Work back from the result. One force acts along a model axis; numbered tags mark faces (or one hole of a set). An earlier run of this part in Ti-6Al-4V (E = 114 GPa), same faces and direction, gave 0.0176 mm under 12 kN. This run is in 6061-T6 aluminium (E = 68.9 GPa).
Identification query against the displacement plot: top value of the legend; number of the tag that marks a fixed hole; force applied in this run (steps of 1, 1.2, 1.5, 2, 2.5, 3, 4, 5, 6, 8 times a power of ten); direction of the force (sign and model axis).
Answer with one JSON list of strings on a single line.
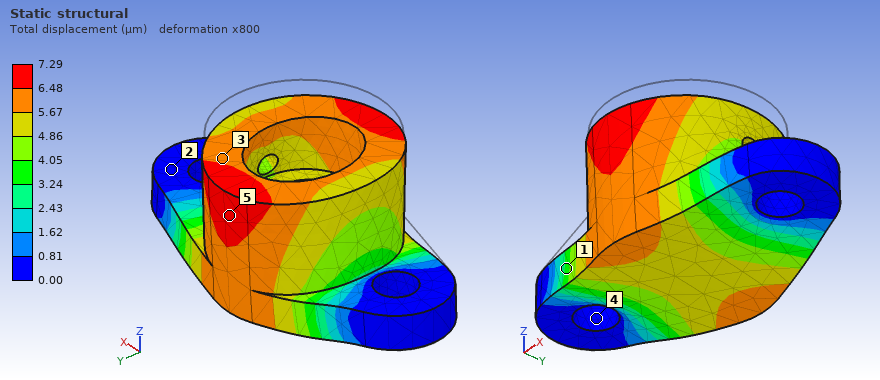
["7.29 µm", "4", "3 kN", "-Z"]
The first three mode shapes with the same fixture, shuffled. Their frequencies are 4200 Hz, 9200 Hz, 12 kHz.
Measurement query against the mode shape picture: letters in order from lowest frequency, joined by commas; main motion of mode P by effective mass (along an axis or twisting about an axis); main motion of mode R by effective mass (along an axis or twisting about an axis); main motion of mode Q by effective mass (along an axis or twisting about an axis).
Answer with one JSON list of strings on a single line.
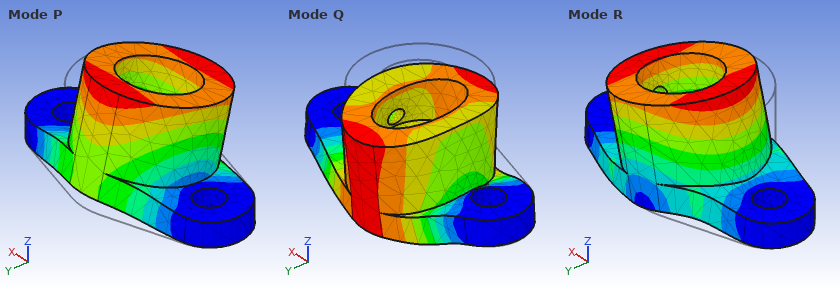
["P, Q, R", "along Y", "along X", "along Z"]
